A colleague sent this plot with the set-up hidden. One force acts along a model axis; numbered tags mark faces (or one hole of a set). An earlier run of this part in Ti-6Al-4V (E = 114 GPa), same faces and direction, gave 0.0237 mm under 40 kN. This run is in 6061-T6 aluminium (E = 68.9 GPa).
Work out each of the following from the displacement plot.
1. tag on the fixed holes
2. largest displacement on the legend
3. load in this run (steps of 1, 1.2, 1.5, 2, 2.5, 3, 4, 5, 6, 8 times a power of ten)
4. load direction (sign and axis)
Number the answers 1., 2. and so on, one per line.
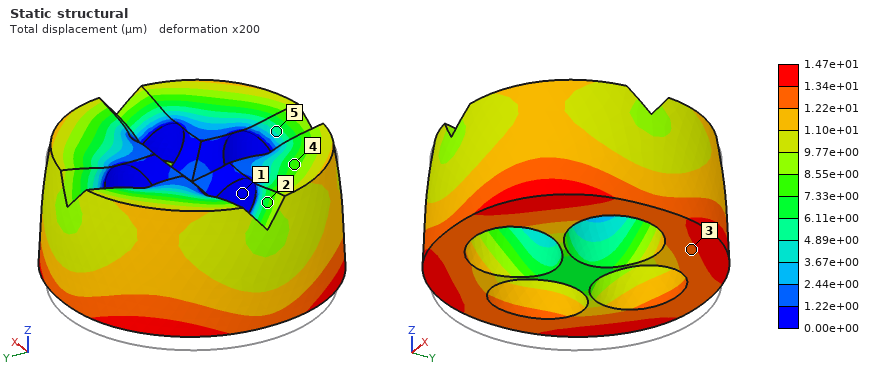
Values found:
1. 1
2. 1.47e+01 µm
3. 15 kN
4. +Z
